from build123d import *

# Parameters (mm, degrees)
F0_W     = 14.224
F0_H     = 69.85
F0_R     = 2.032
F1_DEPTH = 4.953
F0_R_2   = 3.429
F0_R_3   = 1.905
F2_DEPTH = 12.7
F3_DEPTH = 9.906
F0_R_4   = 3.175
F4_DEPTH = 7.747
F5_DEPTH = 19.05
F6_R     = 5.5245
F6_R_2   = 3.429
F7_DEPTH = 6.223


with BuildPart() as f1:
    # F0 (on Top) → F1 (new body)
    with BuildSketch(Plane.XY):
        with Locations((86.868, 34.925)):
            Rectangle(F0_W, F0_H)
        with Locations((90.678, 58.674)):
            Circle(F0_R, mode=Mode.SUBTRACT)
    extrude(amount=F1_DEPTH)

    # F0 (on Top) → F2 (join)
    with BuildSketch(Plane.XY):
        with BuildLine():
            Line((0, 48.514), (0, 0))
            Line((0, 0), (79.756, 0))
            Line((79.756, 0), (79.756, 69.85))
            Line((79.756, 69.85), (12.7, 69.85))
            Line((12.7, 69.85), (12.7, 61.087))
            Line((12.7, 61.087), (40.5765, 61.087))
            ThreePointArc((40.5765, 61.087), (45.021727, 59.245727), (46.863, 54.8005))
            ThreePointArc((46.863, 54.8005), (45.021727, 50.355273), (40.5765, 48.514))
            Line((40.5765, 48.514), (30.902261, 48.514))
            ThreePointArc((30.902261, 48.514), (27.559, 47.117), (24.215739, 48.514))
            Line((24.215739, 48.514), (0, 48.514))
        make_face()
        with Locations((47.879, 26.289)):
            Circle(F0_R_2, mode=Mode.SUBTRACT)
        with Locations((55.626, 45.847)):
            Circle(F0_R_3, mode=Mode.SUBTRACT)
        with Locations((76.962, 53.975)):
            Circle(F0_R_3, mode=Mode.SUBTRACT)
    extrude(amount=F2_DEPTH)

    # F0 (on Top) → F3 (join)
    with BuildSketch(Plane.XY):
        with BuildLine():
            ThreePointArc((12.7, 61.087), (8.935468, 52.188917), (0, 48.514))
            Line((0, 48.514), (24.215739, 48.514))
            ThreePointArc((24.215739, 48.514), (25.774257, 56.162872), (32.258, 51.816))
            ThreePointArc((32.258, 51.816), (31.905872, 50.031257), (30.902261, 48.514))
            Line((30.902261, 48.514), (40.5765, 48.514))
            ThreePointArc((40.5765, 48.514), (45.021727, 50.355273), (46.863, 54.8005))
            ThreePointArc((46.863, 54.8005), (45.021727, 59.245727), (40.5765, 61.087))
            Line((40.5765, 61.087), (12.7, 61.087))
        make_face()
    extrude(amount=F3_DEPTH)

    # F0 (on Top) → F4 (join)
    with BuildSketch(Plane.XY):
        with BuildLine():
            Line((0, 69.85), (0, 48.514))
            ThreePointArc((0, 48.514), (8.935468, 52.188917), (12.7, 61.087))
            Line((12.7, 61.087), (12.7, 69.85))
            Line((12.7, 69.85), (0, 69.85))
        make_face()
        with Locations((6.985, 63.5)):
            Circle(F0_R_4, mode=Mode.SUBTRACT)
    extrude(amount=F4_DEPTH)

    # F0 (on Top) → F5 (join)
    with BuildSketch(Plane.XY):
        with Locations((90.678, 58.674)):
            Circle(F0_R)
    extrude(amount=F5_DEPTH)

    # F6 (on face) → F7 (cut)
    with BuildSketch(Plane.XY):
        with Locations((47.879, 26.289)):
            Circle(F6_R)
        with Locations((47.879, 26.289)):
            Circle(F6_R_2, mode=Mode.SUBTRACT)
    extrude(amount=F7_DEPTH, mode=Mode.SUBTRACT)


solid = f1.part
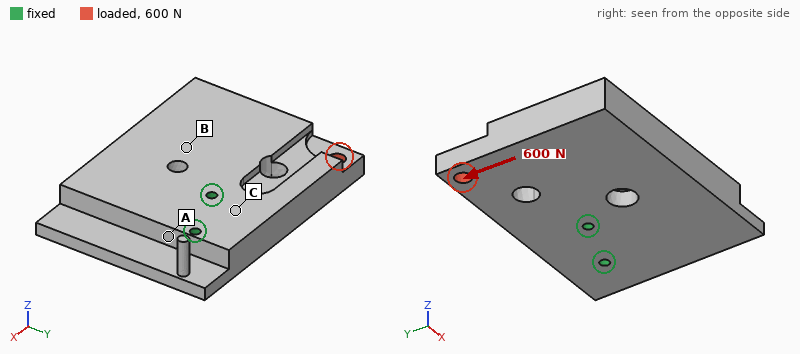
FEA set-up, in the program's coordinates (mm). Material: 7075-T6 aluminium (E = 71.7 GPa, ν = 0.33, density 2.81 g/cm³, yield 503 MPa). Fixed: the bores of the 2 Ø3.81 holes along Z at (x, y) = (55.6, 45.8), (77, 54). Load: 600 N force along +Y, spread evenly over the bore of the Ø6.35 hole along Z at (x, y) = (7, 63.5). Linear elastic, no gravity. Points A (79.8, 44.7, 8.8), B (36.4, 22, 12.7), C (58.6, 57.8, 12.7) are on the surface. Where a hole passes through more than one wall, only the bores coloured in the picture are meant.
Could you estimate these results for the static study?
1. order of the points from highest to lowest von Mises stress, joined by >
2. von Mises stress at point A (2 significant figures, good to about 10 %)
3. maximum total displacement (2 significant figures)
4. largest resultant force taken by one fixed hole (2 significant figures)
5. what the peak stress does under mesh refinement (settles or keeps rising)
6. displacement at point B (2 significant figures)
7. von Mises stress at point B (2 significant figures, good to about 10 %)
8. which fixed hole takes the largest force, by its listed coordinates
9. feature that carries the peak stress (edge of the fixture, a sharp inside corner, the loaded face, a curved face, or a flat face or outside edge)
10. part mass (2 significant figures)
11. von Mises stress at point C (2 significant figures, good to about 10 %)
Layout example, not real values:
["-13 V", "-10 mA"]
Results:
["A > C > B", "6.6 MPa", "15 µm", "1.7 kN", "keeps rising", "6.0 µm", "1.7 MPa", "(55.6, 45.8)", "edge of the fixture", "200 g", "4.3 MPa"]
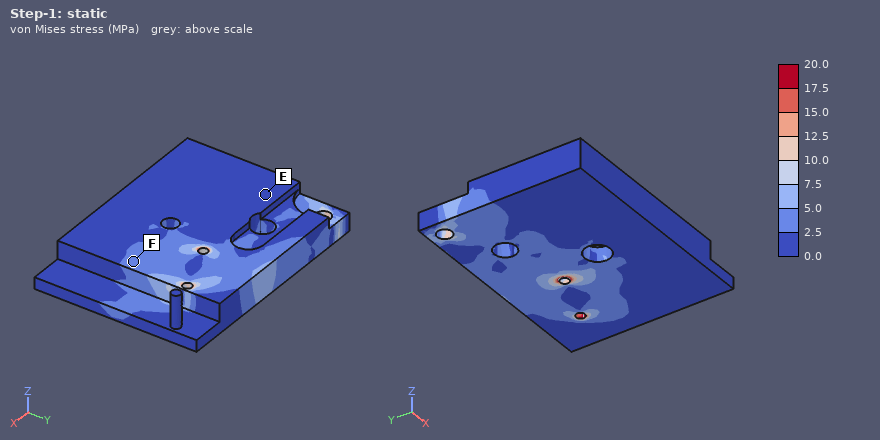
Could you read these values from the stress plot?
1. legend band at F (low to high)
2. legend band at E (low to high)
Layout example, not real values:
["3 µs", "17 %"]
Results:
["2.5 to 5.0 MPa", "0.0 to 2.5 MPa"]
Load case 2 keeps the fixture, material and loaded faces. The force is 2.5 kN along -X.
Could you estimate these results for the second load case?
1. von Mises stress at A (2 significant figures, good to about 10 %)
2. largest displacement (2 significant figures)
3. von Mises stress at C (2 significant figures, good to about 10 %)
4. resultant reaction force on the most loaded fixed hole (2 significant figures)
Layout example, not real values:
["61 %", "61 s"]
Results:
["6.8 MPa", "31 µm", "6.9 MPa", "1.9 kN"]
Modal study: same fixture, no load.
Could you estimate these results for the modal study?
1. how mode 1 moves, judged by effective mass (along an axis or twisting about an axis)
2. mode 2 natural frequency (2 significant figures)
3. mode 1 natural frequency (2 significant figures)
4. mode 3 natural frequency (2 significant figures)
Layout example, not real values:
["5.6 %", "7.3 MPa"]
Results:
["along Z", "3200 Hz", "2200 Hz", "4100 Hz"]
